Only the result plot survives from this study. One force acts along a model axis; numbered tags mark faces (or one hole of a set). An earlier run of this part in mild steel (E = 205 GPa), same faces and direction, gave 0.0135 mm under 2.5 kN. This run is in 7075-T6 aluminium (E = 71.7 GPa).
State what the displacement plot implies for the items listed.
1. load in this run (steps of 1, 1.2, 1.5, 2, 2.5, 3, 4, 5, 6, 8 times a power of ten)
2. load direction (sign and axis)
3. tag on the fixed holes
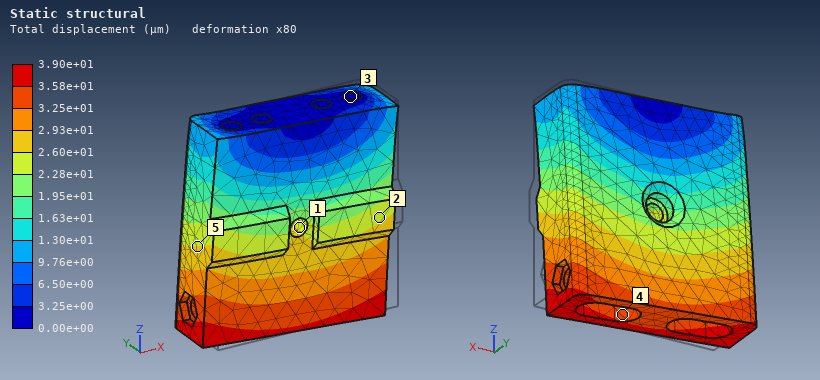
2.5 kN
-X
3
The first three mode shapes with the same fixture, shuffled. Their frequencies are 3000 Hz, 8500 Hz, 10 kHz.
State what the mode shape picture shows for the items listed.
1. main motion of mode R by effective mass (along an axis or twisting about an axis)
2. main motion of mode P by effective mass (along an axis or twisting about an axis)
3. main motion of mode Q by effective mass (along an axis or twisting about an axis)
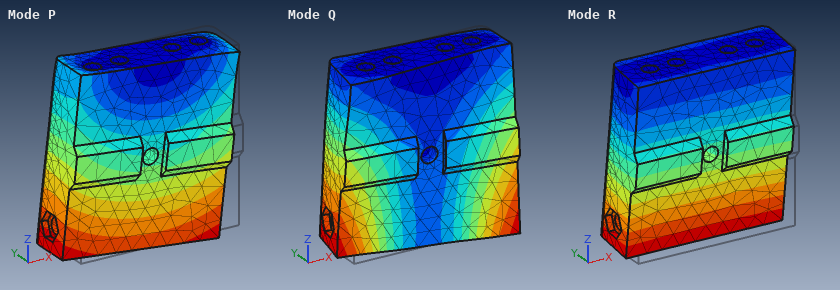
along Y
along X
twisting about Z
